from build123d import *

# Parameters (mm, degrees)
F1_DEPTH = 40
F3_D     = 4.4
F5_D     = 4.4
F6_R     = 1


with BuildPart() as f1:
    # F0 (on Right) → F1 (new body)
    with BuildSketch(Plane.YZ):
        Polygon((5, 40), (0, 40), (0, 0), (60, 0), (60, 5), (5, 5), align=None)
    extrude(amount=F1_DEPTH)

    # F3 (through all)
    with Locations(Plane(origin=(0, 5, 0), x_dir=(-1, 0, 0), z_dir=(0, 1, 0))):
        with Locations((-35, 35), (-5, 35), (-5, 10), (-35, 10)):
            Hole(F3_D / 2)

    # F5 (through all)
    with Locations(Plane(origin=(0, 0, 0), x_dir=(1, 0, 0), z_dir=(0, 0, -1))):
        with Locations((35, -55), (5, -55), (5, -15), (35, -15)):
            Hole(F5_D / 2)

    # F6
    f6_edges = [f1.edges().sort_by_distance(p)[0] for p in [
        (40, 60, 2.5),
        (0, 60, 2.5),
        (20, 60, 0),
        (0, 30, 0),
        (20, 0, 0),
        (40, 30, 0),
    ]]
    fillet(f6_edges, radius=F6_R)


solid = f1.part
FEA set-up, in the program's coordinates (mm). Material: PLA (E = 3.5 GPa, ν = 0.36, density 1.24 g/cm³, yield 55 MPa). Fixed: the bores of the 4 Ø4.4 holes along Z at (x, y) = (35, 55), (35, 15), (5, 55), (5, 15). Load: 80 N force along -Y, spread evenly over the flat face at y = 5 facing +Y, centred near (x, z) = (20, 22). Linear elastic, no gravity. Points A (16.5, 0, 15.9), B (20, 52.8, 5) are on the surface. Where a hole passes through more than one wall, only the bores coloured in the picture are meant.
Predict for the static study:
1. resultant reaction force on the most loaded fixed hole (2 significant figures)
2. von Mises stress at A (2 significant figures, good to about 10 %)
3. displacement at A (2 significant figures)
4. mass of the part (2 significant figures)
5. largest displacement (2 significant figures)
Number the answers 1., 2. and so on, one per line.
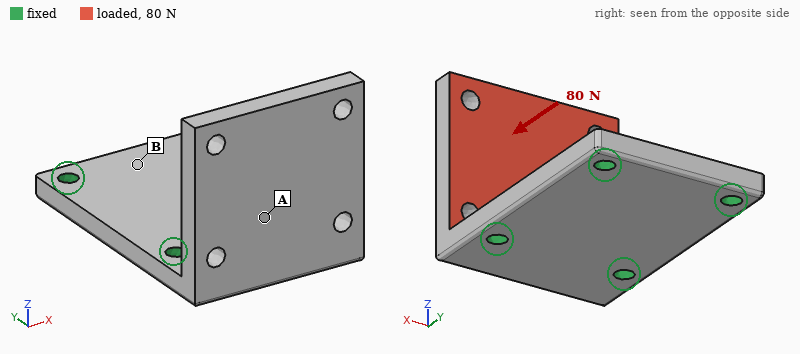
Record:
1. 36 N
2. 3.7 MPa
3. 0.27 mm
4. 23 g
5. 0.84 mm
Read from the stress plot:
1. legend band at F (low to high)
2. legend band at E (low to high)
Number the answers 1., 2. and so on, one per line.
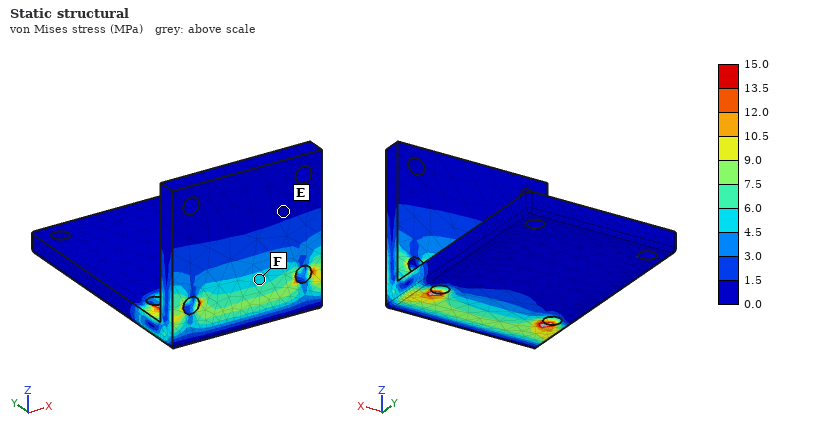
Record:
1. 4.5 to 6.0 MPa
2. 0.0 to 1.5 MPa
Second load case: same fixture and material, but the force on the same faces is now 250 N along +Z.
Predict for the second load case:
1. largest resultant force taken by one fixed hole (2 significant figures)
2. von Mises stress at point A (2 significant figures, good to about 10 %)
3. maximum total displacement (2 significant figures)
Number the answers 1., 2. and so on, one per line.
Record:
1. 130 N
2. 1.9 MPa
3. 0.16 mm
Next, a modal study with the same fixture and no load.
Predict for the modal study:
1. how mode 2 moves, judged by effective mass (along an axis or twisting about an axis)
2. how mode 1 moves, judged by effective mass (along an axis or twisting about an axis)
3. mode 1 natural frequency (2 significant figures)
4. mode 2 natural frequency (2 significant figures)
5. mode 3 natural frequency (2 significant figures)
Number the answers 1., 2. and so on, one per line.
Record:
1. along X
2. along Y
3. 660 Hz
4. 1600 Hz
5. 2200 Hz
